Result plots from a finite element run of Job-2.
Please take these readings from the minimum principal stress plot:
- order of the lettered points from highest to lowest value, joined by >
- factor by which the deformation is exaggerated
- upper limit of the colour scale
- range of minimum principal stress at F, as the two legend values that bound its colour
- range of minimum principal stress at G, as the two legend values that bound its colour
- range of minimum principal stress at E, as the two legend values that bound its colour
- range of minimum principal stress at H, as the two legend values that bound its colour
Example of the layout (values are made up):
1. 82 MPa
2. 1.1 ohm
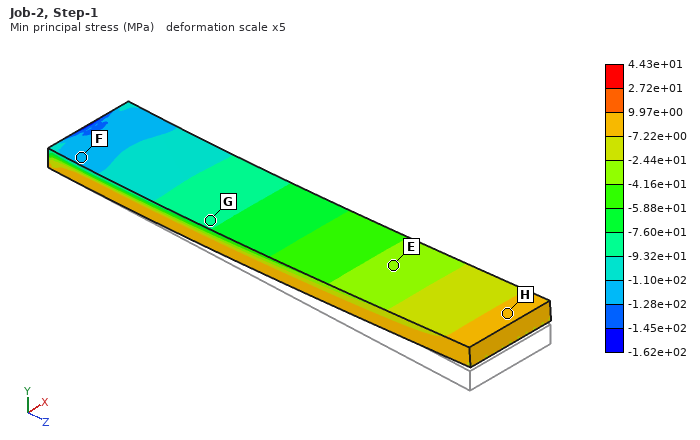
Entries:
1. H > E > G > F
2. 5
3. 4.43e+01 MPa
4. -1.28e+02 to -1.10e+02 MPa
5. -9.32e+01 to -7.60e+01 MPa
6. -4.16e+01 to -2.44e+01 MPa
7. -7.22e+00 to 9.97e+00 MPa
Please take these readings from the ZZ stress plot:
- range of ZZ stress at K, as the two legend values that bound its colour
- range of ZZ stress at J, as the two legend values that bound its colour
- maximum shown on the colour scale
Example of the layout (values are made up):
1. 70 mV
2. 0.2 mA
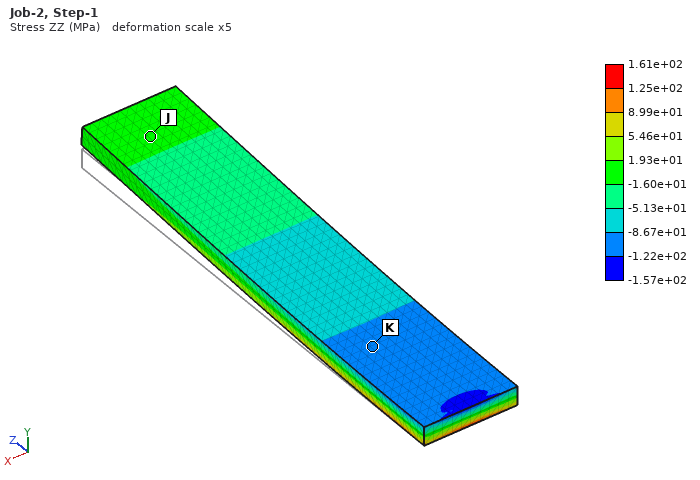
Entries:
1. -1.22e+02 to -8.67e+01 MPa
2. -1.60e+01 to 1.93e+01 MPa
3. 1.61e+02 MPa
